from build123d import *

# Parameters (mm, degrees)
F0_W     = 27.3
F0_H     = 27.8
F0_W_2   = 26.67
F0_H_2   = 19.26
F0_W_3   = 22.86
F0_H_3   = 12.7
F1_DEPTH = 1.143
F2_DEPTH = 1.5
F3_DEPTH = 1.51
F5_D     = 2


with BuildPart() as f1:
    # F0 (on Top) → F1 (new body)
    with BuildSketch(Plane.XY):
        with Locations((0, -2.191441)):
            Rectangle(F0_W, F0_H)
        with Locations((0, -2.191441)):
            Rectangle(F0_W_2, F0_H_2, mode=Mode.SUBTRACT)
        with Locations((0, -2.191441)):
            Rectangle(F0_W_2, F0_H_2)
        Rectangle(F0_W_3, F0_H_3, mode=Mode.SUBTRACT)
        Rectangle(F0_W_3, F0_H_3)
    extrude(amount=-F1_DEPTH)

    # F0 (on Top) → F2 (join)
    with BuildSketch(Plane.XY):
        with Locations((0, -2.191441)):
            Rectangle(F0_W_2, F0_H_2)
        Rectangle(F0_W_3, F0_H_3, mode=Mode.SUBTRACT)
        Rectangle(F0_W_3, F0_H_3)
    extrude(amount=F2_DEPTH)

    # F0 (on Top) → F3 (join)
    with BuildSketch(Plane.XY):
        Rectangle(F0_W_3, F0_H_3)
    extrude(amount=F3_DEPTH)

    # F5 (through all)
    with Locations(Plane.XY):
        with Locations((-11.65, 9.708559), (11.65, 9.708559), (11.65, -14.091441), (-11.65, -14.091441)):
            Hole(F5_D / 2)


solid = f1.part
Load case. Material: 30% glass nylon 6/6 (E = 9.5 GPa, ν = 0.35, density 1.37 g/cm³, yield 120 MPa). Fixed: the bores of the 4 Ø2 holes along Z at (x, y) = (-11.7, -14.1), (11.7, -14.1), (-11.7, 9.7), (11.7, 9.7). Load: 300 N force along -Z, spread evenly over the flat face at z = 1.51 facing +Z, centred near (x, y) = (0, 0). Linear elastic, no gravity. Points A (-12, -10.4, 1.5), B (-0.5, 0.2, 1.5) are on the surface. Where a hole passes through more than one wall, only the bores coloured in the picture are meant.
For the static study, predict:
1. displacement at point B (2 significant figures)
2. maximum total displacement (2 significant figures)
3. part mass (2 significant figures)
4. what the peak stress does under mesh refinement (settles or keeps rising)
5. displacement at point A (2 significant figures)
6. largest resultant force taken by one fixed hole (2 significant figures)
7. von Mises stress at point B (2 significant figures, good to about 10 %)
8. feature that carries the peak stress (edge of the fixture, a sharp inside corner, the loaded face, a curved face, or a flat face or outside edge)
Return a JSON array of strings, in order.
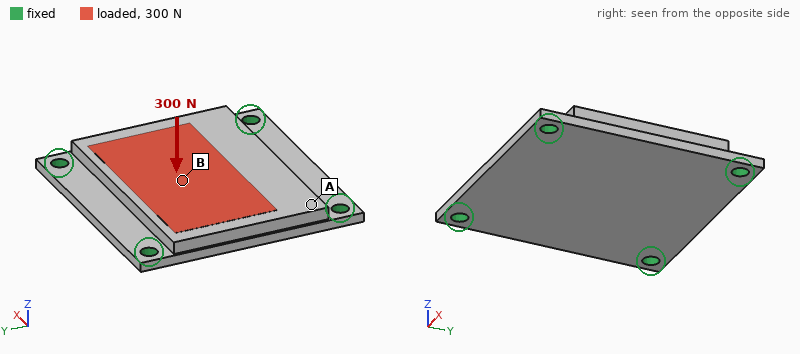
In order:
["0.16 mm", "0.16 mm", "2.2 g", "keeps rising", "0.038 mm", "150 N", "27 MPa", "edge of the fixture"]
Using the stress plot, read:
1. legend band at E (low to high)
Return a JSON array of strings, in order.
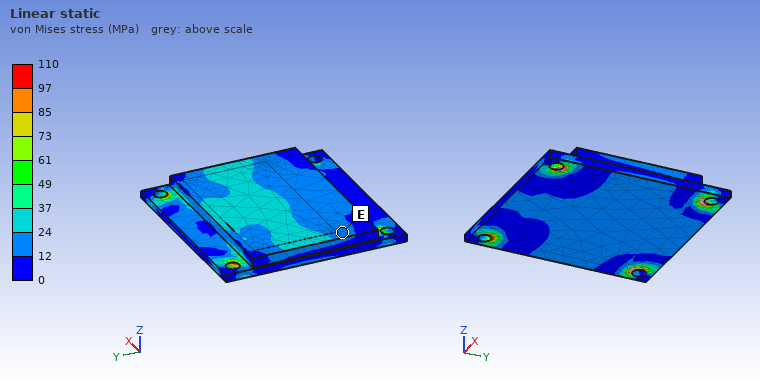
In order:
["12 to 24 MPa"]
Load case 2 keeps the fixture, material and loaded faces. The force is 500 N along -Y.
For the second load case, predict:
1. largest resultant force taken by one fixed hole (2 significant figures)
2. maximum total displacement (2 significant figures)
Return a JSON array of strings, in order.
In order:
["140 N", "34 µm"]
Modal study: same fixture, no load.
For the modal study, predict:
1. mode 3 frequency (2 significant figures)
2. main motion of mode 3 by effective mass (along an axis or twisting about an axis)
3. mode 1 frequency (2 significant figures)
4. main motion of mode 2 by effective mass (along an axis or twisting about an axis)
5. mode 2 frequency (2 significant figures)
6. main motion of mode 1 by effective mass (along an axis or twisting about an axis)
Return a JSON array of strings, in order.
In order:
["10 kHz", "twisting about Y", "5900 Hz", "twisting about X", "9700 Hz", "along Z"]
